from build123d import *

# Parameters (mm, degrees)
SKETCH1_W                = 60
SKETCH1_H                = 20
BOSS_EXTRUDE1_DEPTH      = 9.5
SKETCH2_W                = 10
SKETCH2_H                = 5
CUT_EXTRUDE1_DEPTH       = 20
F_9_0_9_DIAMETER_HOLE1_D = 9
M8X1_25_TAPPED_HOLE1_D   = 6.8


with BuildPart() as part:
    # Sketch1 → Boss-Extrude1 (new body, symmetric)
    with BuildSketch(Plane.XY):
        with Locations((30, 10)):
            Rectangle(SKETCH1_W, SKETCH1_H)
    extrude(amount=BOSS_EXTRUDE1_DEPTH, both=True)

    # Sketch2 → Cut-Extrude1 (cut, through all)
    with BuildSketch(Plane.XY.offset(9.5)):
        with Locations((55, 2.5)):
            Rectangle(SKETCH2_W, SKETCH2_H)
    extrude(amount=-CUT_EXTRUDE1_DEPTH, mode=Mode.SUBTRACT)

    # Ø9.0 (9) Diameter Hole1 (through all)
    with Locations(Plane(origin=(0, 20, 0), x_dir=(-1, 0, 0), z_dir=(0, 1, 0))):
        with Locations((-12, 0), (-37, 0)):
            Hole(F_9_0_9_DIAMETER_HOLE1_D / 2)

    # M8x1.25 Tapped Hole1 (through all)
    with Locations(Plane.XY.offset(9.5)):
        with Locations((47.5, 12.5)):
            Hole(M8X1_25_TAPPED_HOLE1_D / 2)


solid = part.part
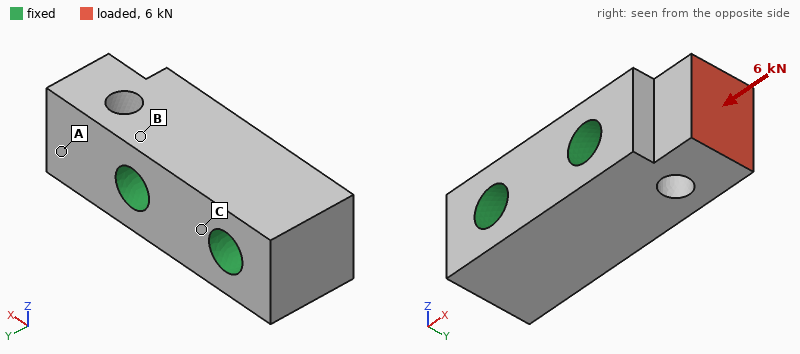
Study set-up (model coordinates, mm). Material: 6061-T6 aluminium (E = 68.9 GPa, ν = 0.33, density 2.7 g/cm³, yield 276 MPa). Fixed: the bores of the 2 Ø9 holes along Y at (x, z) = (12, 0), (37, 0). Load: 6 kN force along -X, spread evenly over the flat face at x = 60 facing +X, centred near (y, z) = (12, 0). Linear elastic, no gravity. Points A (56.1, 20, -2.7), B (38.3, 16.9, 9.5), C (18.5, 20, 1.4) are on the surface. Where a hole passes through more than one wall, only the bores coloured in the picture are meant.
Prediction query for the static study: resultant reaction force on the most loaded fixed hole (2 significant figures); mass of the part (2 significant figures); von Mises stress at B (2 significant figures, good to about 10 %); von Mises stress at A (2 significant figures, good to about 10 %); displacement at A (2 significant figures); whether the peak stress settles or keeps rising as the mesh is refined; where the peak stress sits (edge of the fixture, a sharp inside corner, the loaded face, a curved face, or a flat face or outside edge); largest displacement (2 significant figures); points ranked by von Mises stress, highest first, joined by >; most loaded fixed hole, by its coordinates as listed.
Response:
5.7 kN
50 g
16 MPa
26 MPa
9.3 µm
keeps rising
edge of the fixture
11 µm
A > B > C
(37, 0)
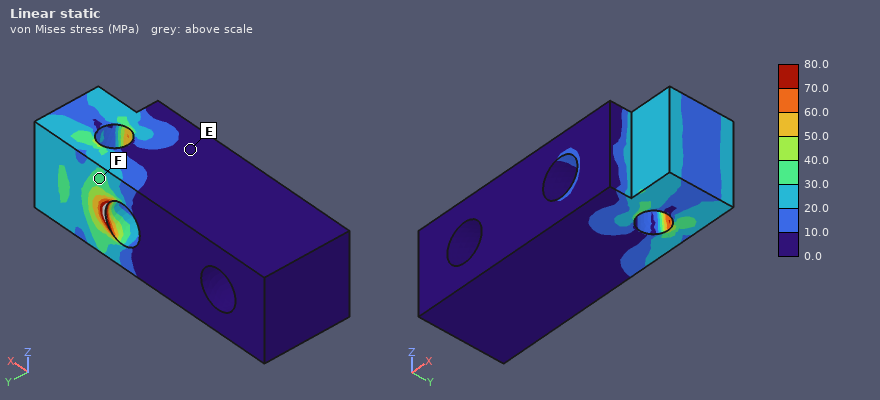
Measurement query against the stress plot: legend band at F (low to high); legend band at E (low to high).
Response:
30.0 to 40.0 MPa
0.0 to 10.0 MPa
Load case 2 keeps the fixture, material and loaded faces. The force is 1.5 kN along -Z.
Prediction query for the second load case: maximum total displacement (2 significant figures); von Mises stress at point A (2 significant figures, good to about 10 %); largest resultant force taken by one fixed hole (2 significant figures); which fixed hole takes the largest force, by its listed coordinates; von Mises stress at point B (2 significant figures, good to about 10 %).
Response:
20 µm
16 MPa
1.8 kN
(37, 0)
20 MPa
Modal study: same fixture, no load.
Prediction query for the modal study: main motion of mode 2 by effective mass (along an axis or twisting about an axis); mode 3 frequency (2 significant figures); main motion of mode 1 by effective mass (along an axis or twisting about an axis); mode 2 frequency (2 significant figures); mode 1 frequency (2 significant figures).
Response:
along Y
35 kHz
along Z
24 kHz
20 kHz
